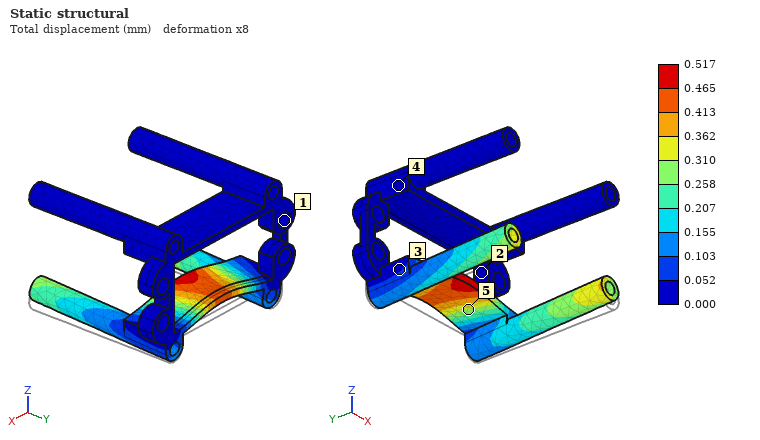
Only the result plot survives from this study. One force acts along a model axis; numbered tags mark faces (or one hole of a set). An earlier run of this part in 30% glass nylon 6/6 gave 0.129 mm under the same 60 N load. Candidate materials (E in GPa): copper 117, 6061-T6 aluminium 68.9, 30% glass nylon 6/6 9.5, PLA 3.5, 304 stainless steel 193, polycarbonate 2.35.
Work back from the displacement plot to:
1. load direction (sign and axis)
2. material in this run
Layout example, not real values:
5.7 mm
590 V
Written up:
+Z
polycarbonate
